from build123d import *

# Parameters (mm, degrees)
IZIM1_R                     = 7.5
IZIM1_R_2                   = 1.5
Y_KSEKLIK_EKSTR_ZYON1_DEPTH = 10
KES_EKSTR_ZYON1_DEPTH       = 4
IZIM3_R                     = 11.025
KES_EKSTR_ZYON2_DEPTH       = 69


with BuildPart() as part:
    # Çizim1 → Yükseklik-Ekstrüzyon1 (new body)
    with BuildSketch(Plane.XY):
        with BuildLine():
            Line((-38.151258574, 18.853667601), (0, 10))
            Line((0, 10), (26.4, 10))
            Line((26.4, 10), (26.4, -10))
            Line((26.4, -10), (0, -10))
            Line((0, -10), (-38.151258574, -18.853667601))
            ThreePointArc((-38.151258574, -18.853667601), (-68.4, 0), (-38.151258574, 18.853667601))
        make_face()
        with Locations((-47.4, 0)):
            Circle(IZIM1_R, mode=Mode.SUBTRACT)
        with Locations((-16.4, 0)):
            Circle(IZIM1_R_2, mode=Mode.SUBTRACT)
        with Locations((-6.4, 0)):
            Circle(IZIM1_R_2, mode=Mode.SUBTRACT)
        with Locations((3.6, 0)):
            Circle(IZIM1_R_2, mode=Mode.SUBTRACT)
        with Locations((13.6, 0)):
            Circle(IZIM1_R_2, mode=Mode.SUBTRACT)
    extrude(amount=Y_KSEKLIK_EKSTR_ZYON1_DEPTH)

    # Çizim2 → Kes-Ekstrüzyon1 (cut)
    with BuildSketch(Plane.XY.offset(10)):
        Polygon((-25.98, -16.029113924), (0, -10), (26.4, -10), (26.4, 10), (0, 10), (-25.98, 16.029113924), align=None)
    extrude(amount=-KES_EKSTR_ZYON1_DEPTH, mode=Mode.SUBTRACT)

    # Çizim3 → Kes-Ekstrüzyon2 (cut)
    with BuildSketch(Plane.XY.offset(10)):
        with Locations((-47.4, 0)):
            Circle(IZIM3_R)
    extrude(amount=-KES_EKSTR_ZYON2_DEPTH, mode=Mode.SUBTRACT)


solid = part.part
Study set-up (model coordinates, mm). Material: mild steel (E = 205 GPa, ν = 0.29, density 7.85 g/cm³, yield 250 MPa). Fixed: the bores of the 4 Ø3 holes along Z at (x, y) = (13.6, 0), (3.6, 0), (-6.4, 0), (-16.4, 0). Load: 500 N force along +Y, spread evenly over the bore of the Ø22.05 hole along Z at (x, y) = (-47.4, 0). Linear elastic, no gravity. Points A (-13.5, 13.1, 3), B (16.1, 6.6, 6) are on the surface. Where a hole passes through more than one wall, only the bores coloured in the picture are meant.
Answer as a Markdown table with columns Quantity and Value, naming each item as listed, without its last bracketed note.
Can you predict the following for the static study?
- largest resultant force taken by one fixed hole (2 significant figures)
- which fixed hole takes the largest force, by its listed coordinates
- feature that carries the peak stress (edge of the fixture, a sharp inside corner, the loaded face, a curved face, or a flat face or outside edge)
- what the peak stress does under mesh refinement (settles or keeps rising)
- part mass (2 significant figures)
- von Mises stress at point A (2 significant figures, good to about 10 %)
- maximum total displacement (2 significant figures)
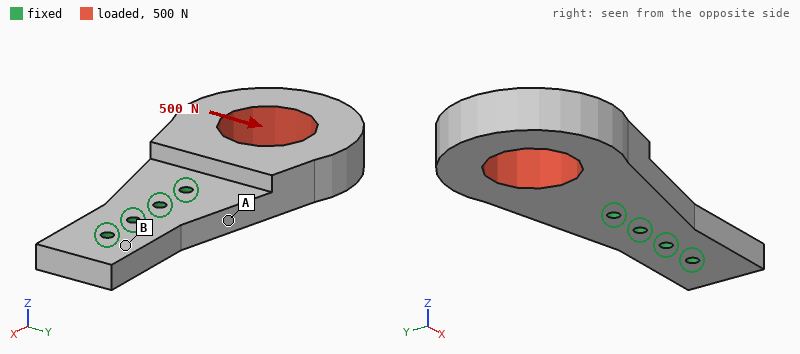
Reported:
| Quantity | Value |
|---|---|
| largest resultant force taken by one fixed hole | 1.3 kN |
| which fixed hole takes the largest force, by its listed coordinates | (-16.4, 0) |
| feature that carries the peak stress | edge of the fixture |
| what the peak stress does under mesh refinement | keeps rising |
| part mass | 140 g |
| von Mises stress at point A | 21 MPa |
| maximum total displacement | 13 µm |
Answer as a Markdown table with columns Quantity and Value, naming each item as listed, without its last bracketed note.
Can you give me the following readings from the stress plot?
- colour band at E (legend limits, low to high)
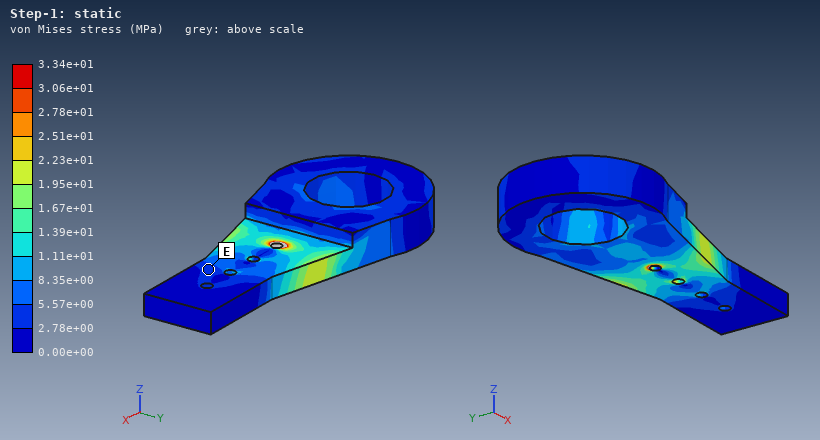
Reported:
| Quantity | Value |
|---|---|
| colour band at E | 2.78e+00 to 5.57e+00 MPa |
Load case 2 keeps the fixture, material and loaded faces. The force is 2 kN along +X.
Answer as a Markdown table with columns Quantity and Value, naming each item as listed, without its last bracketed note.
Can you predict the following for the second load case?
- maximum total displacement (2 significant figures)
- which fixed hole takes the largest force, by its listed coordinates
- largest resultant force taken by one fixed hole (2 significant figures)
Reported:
| Quantity | Value |
|---|---|
| maximum total displacement | 24 µm |
| which fixed hole takes the largest force, by its listed coordinates | (-16.4, 0) |
| largest resultant force taken by one fixed hole | 1.2 kN |
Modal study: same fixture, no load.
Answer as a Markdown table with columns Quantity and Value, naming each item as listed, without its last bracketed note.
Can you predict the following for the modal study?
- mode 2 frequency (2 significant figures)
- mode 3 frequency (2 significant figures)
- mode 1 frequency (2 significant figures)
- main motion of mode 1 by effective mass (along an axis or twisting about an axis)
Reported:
| Quantity | Value |
|---|---|
| mode 2 frequency | 3900 Hz |
| mode 3 frequency | 4100 Hz |
| mode 1 frequency | 1600 Hz |
| main motion of mode 1 by effective mass | along Z |
